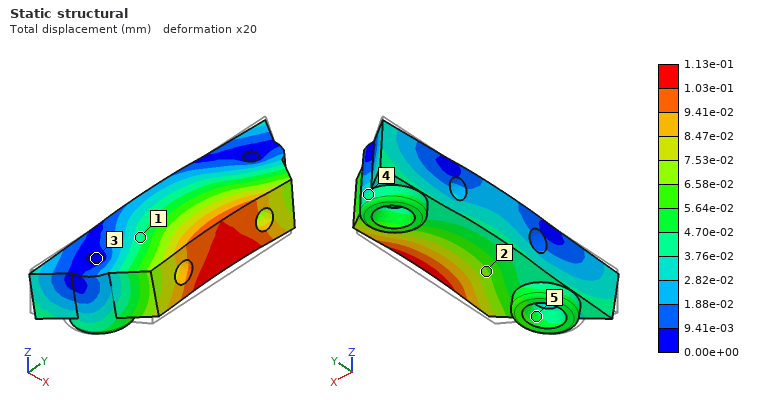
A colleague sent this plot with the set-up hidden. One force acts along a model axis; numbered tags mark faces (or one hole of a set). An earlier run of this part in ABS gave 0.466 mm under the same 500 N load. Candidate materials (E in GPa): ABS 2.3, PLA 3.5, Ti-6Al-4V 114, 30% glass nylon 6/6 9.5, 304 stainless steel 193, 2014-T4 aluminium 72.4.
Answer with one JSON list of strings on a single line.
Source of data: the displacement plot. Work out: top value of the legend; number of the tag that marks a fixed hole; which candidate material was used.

["1.13e-01 mm", "3", "30% glass nylon 6/6"]
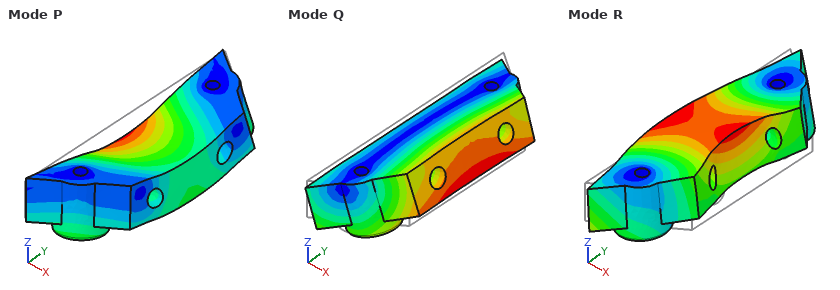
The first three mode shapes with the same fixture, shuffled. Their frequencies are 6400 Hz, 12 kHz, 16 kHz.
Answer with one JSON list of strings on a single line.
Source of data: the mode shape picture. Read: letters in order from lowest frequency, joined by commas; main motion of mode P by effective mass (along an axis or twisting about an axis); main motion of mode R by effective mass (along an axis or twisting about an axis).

["Q, P, R", "along Z", "along X"]
